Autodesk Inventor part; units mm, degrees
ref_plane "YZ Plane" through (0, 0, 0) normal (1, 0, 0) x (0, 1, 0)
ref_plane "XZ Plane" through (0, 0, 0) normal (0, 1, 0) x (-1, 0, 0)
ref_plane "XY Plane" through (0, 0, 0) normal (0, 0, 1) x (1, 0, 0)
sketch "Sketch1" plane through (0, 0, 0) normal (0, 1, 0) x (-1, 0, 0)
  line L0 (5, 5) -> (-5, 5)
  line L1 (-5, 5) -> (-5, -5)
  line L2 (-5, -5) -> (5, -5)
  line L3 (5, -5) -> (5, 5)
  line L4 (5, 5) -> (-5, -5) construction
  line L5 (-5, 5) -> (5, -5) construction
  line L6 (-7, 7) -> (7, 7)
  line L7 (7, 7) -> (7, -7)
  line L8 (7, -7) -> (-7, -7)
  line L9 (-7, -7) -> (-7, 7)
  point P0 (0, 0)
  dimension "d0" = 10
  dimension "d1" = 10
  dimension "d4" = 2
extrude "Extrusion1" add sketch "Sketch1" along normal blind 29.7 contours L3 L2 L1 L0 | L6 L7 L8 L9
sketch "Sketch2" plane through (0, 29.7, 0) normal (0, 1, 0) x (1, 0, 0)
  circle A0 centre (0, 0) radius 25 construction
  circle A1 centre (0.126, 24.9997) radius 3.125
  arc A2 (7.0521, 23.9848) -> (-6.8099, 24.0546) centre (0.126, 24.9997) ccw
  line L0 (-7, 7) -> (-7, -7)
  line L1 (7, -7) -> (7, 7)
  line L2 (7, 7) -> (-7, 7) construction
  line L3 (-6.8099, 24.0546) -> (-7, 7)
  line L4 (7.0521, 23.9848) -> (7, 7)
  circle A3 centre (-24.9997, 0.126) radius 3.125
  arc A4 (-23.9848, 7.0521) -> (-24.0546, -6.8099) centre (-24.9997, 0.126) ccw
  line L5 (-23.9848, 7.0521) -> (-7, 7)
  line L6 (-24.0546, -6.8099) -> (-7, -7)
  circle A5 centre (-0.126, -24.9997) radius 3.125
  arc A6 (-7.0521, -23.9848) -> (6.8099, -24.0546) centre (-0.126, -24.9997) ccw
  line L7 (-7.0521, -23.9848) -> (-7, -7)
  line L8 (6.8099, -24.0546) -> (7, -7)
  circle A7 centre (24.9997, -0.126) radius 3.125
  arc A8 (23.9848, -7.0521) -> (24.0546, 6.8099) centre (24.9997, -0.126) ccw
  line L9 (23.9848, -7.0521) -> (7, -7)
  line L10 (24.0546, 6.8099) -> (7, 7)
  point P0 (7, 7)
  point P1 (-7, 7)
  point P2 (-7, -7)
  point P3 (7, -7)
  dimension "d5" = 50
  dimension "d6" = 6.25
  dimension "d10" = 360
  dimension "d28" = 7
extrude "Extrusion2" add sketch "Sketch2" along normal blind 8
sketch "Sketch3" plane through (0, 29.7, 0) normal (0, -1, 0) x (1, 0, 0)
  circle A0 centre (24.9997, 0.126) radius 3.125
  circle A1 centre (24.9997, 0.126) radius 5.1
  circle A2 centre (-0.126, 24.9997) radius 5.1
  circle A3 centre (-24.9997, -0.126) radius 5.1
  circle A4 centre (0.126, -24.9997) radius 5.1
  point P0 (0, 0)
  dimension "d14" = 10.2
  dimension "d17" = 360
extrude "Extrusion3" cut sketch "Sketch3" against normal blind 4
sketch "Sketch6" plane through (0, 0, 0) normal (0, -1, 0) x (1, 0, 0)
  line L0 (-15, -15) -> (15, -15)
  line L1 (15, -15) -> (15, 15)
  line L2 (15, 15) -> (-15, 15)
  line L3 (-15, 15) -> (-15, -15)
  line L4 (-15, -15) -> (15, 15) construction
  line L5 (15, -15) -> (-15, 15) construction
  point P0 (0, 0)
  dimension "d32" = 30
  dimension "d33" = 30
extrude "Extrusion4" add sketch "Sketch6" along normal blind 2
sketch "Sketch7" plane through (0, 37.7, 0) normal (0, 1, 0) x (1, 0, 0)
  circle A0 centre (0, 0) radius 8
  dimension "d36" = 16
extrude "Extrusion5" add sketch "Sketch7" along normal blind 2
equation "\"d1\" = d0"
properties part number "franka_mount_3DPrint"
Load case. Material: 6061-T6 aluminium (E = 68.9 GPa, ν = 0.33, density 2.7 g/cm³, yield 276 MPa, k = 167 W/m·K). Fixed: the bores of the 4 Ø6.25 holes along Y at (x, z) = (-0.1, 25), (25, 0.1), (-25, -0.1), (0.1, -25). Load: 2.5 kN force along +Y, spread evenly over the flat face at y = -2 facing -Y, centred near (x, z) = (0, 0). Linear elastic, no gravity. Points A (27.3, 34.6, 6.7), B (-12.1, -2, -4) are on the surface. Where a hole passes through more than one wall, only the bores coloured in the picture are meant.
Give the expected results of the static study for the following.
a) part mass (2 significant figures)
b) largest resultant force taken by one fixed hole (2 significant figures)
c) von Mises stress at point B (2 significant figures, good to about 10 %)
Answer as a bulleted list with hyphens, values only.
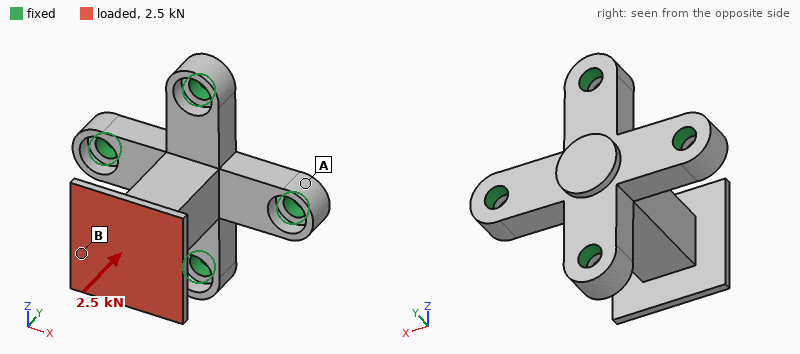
- 49 g
- 850 N
- 66 MPa
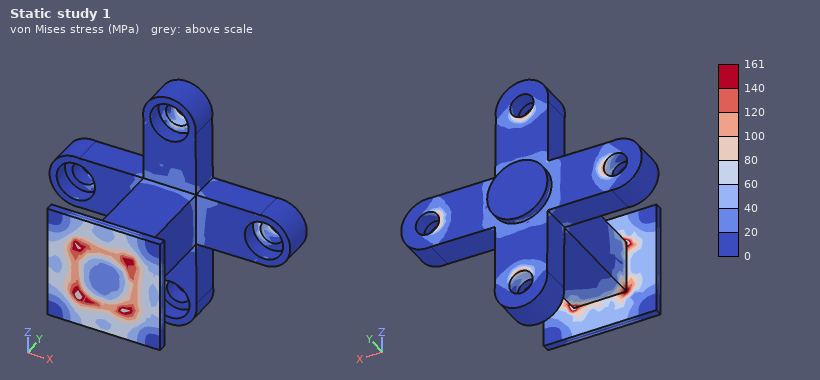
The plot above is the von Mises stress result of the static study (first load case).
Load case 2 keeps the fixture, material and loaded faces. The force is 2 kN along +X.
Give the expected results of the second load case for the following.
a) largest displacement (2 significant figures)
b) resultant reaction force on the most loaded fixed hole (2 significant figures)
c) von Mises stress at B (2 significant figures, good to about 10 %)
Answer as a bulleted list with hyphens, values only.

- 0.26 mm
- 2.1 kN
- 16 MPa
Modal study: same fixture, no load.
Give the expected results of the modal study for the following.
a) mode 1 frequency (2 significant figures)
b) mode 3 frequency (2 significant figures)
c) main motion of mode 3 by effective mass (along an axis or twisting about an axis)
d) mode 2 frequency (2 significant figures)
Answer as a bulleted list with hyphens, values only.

- 5000 Hz
- 10 kHz
- along Y
- 5000 Hz
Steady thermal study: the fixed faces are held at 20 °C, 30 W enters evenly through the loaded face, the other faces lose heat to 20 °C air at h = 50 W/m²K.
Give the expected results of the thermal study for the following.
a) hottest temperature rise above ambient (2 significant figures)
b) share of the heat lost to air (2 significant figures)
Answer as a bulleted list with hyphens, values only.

- 42 K
- 14 %
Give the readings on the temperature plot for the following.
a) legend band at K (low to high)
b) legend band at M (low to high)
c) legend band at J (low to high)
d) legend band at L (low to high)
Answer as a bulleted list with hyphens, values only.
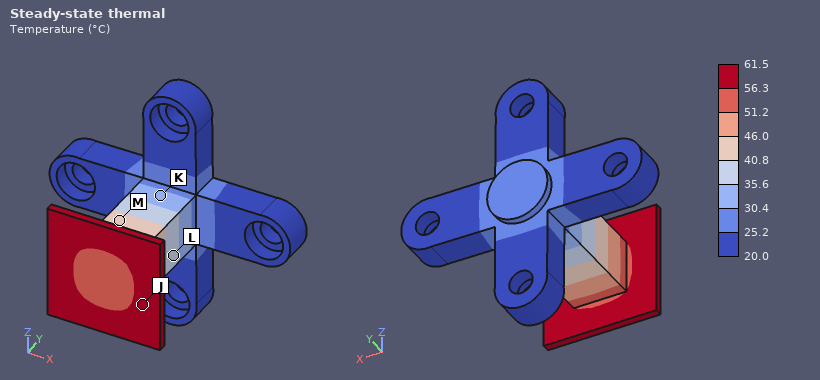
- 30.4 to 35.6 °C
- 40.8 to 46.0 °C
- 56.3 to 61.5 °C
- 35.6 to 40.8 °C
